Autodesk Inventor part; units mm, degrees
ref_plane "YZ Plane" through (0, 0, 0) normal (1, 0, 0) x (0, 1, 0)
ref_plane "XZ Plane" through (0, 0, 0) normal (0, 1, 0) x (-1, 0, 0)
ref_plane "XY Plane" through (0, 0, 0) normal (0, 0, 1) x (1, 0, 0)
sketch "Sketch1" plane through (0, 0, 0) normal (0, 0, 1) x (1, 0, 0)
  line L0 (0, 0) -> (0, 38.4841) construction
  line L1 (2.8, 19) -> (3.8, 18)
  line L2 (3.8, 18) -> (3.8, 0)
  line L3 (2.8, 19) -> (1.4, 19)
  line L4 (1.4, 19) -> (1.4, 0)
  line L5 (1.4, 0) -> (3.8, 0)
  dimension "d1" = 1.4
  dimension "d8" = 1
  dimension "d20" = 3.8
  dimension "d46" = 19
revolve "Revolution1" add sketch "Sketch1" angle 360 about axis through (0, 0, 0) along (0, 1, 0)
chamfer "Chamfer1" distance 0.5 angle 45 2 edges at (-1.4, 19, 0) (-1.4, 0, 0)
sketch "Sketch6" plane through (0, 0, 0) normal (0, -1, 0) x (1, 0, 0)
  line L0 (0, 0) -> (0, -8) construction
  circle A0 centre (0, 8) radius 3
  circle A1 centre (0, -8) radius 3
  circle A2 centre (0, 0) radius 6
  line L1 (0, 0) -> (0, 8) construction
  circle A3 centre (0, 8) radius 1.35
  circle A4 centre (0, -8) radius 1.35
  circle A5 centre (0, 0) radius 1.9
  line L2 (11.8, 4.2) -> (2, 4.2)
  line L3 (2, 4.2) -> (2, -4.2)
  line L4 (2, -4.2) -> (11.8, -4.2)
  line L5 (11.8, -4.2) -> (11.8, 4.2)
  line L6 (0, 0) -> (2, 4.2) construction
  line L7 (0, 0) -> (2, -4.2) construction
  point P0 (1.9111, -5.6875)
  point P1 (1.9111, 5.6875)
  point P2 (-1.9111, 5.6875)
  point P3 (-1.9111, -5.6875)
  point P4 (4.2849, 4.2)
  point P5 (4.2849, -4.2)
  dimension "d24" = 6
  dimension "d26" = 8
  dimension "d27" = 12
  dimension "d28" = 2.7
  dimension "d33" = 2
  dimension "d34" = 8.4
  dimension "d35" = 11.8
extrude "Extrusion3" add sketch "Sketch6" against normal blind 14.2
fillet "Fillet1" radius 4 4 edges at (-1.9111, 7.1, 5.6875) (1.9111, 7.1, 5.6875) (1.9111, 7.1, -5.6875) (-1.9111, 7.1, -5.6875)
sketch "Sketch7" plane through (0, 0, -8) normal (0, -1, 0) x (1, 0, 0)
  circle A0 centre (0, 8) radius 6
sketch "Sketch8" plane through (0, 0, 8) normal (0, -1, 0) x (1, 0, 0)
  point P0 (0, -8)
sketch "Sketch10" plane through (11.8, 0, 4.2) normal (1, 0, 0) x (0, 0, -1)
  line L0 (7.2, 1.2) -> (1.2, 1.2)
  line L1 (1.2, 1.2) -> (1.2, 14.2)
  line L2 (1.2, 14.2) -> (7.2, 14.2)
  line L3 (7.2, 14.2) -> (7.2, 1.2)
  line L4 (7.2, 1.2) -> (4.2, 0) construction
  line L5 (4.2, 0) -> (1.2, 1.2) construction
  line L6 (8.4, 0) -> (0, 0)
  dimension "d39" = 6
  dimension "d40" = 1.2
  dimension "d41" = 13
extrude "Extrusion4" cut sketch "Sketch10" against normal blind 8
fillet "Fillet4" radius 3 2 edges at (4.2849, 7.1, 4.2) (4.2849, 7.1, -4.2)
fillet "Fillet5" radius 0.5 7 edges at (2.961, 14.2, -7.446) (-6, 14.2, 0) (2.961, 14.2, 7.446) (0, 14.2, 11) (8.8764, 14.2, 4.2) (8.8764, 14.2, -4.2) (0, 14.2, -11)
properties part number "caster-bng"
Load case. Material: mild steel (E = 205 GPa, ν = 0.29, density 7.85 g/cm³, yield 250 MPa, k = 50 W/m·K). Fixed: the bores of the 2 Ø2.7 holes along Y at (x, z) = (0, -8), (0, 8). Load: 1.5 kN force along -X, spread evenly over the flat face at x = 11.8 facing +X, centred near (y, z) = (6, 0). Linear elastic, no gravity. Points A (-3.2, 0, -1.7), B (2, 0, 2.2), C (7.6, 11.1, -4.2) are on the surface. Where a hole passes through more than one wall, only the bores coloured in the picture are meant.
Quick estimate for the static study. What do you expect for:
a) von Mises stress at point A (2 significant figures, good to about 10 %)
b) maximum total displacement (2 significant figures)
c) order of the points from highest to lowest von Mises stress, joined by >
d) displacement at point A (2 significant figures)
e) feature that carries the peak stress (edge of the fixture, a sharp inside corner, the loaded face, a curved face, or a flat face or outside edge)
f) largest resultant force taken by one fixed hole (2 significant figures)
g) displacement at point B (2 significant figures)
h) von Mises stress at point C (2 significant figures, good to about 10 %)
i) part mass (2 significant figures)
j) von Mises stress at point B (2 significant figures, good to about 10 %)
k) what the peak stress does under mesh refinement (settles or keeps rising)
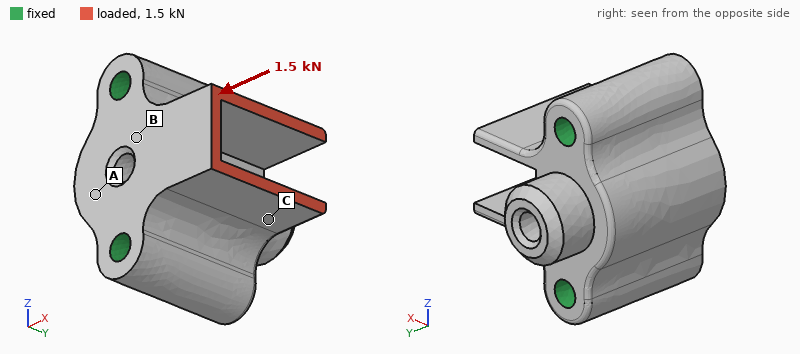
8.9 MPa
3.1 µm
C > B > A
0.67 µm
edge of the fixture
760 N
1.00 µm
38 MPa
20 g
24 MPa
keeps rising
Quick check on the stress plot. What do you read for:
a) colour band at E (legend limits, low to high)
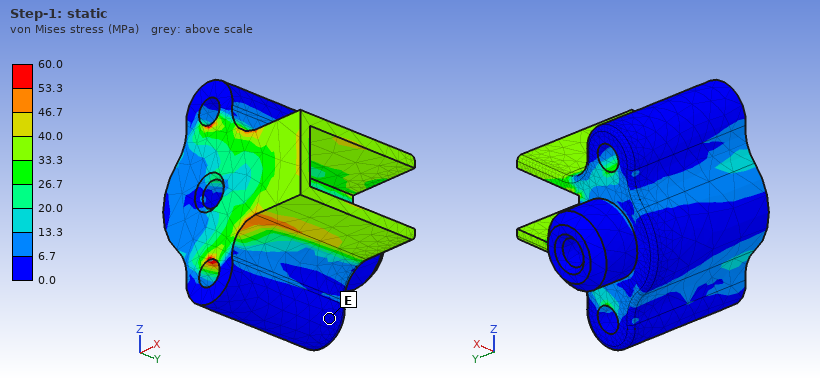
0.0 to 6.7 MPa
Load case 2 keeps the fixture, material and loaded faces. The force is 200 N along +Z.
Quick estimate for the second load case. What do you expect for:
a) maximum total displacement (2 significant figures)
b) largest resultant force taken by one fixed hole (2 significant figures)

22 µm
190 N
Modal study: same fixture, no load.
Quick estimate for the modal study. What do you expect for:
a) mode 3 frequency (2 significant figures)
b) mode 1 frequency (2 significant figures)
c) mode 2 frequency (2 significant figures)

43 kHz
21 kHz
21 kHz
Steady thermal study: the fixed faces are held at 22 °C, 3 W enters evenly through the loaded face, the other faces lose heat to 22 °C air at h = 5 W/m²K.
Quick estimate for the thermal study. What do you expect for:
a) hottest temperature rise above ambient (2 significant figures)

14 K
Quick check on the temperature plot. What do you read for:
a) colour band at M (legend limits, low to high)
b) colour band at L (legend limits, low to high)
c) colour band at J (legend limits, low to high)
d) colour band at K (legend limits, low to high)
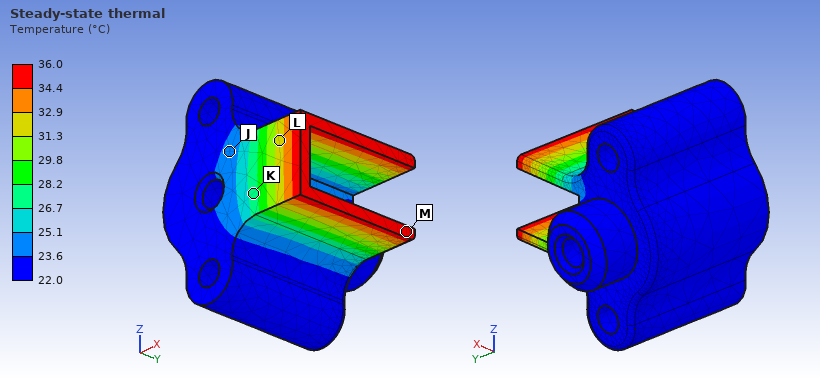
34.4 to 36.0 °C
31.3 to 32.9 °C
23.6 to 25.1 °C
26.7 to 28.2 °C
